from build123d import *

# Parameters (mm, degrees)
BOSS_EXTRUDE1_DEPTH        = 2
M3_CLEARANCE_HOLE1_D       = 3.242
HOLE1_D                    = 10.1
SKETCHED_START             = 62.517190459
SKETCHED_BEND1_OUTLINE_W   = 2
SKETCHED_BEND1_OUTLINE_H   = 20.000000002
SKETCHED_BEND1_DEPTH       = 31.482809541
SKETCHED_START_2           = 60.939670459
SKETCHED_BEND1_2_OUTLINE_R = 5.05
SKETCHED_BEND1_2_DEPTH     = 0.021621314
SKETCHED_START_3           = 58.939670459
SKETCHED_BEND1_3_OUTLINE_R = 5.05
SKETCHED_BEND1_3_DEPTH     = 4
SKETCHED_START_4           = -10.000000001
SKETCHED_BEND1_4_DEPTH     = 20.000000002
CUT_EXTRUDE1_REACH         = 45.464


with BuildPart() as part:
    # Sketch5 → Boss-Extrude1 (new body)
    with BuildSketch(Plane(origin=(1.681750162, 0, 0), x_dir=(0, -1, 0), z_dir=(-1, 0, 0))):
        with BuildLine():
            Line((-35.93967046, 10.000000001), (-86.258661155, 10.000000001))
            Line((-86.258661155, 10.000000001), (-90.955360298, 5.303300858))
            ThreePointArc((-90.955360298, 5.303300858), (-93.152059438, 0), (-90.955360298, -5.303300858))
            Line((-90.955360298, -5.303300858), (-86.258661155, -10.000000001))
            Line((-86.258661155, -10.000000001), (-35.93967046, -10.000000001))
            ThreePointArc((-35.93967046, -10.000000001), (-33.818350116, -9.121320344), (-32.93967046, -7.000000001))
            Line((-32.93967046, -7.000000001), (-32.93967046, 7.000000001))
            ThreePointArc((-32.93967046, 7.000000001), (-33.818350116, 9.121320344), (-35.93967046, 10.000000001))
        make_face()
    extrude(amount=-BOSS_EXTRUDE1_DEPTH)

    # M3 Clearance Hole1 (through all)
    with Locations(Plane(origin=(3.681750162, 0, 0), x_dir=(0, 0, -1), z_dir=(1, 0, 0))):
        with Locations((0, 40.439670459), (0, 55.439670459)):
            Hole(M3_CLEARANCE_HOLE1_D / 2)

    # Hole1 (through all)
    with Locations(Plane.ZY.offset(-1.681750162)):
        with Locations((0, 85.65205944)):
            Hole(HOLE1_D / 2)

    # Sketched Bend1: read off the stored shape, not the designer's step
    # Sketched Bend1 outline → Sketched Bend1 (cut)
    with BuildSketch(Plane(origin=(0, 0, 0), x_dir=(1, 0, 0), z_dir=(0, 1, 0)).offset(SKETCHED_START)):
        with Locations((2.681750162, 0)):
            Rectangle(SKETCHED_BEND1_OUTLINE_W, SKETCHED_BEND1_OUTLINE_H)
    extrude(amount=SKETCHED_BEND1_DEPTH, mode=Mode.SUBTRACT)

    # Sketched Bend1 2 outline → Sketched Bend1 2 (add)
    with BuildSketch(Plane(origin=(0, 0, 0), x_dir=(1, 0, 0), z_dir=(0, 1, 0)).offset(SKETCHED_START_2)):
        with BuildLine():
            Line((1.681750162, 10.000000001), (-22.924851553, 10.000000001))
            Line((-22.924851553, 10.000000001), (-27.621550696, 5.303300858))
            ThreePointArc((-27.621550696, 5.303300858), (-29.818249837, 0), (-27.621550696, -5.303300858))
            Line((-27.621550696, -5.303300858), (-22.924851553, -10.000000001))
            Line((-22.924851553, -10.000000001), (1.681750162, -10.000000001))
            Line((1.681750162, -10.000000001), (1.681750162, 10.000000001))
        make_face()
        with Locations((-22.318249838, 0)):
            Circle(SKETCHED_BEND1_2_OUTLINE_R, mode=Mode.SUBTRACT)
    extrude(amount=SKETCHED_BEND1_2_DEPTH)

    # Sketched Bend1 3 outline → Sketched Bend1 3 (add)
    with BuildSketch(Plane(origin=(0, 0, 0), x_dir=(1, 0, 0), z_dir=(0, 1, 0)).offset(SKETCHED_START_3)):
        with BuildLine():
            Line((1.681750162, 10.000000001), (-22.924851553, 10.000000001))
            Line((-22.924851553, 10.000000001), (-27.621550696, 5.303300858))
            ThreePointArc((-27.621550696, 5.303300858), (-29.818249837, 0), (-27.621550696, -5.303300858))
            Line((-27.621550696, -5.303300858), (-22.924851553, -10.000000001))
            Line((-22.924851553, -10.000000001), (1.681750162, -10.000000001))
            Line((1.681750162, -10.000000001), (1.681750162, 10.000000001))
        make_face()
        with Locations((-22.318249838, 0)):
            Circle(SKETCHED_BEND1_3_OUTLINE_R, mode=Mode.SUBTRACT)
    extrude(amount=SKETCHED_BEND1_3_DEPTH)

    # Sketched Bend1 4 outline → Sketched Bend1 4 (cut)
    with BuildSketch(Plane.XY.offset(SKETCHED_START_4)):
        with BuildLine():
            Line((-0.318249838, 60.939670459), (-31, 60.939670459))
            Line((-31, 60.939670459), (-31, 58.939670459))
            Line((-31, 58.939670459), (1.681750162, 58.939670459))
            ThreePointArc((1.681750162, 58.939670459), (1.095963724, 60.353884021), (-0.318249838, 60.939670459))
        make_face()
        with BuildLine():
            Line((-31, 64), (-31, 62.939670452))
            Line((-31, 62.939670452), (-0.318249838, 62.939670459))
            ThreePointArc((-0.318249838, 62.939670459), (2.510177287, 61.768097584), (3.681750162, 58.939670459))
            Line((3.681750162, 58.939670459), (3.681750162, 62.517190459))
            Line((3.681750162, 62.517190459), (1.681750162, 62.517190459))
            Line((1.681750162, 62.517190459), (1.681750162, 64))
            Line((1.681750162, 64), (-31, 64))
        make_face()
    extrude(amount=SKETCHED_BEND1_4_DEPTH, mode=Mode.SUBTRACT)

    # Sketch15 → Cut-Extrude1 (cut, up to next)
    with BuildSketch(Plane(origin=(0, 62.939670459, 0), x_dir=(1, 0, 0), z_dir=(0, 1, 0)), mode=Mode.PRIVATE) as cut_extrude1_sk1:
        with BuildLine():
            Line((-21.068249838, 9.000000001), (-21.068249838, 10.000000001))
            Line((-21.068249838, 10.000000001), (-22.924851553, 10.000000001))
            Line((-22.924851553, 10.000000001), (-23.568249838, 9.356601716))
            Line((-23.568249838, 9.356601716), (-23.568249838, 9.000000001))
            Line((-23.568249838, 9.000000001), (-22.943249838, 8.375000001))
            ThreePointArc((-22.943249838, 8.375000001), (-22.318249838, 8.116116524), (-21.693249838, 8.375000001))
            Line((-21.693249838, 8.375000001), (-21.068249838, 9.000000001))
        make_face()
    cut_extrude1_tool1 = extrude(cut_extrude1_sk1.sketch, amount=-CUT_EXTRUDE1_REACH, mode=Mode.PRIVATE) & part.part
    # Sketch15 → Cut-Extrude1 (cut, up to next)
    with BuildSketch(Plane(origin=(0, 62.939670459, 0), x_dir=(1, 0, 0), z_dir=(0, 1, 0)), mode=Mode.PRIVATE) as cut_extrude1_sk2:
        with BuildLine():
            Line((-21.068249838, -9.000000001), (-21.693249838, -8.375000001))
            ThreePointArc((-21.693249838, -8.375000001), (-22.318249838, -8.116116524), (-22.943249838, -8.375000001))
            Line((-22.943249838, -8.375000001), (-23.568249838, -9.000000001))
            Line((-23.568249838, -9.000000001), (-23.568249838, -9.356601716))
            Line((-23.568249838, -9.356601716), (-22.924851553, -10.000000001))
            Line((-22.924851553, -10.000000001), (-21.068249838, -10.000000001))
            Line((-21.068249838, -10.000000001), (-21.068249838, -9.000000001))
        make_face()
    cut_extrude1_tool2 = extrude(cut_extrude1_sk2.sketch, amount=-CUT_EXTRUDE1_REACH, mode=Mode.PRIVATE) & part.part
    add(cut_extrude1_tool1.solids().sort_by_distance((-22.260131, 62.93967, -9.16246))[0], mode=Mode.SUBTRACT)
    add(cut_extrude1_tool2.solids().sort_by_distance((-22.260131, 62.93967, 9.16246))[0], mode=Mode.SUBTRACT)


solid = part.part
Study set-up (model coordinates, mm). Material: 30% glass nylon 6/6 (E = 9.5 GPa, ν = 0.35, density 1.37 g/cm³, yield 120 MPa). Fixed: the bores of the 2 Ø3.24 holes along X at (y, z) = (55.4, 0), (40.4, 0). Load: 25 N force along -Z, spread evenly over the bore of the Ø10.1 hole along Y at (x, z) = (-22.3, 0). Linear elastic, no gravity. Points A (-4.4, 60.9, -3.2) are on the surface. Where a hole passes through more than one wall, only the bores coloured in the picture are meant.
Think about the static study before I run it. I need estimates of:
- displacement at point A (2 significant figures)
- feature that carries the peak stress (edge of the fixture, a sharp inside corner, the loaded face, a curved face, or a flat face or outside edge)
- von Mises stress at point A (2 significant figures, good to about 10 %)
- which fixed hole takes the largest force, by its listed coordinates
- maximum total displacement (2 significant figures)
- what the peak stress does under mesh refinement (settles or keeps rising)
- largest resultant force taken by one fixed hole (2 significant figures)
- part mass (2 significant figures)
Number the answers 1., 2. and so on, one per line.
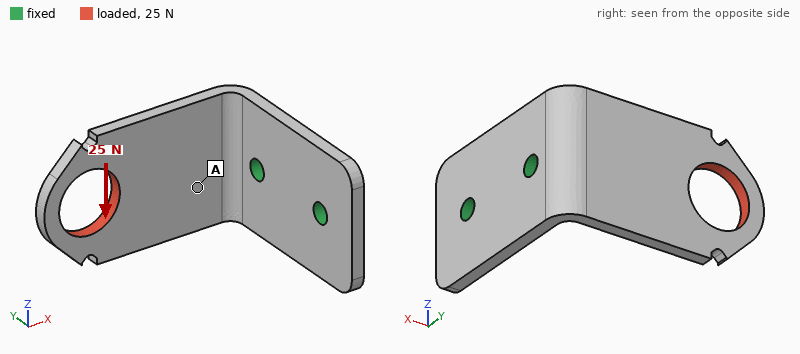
1. 0.13 mm
2. edge of the fixture
3. 7.4 MPa
4. (55.4, 0)
5. 0.54 mm
6. keeps rising
7. 32 N
8. 2.9 g
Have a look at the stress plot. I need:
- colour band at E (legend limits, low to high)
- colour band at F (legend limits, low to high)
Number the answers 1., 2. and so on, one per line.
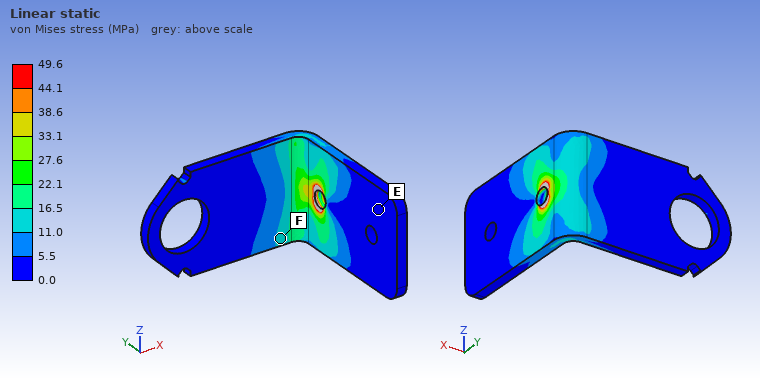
1. 0.0 to 5.5 MPa
2. 11.0 to 16.5 MPa
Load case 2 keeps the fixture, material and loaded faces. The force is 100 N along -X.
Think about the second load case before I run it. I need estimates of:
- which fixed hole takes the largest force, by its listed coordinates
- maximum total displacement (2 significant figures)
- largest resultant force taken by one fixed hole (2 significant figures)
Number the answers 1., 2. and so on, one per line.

1. (55.4, 0)
2. 0.55 mm
3. 110 N
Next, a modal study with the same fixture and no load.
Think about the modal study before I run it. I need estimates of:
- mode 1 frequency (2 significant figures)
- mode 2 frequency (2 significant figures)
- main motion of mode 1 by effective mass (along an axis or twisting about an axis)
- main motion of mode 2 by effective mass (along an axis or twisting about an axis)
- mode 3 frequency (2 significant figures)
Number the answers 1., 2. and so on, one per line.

1. 890 Hz
2. 1500 Hz
3. along Y
4. along Z
5. 3300 Hz
